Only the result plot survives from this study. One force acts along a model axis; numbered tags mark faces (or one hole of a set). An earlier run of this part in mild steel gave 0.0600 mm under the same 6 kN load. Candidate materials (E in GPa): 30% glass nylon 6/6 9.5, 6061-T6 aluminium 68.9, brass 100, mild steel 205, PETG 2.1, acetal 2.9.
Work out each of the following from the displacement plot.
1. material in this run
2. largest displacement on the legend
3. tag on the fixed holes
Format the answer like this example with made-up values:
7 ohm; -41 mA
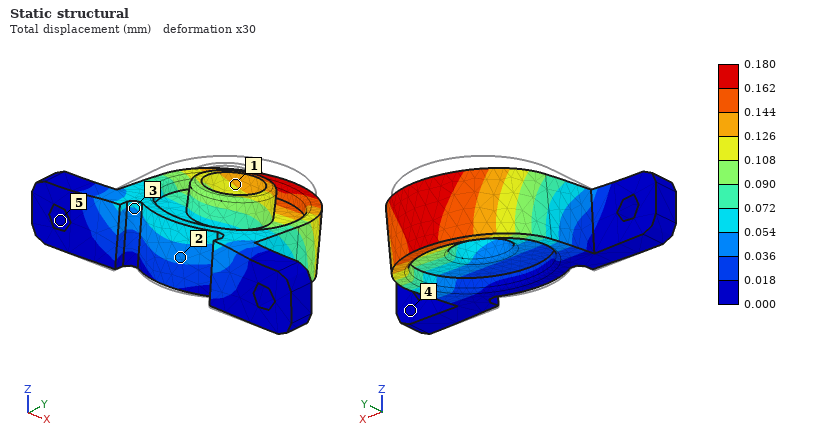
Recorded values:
6061-T6 aluminium; 0.180 mm; 5
